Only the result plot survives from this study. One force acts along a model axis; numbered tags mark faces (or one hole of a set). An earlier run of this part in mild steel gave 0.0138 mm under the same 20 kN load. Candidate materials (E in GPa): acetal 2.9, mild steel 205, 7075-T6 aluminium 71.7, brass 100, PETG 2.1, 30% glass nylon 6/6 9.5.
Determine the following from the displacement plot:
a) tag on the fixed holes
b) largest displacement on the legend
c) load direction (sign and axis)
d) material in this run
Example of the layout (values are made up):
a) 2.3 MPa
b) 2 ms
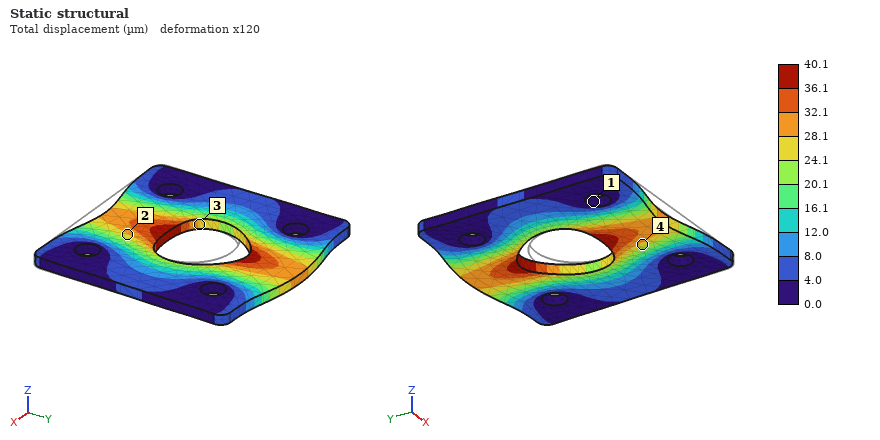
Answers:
a) 1
b) 40.1 µm
c) +Y
d) 7075-T6 aluminium
